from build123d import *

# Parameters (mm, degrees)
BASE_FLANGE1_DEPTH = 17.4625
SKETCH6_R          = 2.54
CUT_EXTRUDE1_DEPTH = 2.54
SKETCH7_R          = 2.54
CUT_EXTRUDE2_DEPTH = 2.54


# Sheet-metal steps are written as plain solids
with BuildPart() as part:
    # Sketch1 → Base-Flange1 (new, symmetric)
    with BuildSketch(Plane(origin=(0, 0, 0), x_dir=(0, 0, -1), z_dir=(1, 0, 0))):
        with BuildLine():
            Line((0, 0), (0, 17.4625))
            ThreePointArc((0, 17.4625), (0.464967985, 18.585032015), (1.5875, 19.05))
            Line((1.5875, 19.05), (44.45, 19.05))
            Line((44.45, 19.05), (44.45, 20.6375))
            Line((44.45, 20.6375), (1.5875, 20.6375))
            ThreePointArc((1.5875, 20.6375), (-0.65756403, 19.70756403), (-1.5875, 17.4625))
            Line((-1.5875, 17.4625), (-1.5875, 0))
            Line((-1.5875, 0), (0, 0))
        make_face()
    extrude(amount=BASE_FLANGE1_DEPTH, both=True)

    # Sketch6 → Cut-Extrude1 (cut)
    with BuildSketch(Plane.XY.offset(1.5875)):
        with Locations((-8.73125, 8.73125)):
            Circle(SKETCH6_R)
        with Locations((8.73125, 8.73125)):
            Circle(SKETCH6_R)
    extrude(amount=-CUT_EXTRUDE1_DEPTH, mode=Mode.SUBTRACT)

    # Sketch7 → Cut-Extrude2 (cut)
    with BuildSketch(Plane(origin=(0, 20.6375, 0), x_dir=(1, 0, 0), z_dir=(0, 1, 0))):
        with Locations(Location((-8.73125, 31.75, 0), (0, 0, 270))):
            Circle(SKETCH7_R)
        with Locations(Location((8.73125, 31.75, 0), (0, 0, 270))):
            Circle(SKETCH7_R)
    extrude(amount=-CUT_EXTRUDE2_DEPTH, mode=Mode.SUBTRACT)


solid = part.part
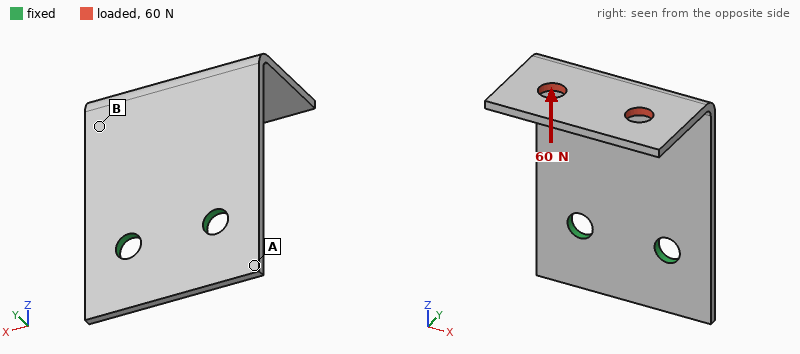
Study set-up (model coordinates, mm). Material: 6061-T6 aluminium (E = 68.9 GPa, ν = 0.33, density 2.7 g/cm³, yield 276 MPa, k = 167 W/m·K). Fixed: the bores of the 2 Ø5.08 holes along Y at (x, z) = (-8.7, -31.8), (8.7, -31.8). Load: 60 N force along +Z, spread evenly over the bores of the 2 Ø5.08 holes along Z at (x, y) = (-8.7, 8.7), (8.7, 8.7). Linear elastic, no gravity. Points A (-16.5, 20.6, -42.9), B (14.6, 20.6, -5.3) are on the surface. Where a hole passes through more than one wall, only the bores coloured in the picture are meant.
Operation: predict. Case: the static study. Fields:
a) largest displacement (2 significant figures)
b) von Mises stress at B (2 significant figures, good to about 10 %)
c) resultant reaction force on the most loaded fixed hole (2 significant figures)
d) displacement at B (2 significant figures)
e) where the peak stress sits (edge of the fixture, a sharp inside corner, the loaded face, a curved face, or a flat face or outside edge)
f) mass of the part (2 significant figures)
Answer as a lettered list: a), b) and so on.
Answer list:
a) 0.67 mm
b) 43 MPa
c) 30 N
d) 0.24 mm
e) a flat face or outside edge
f) 9.2 g
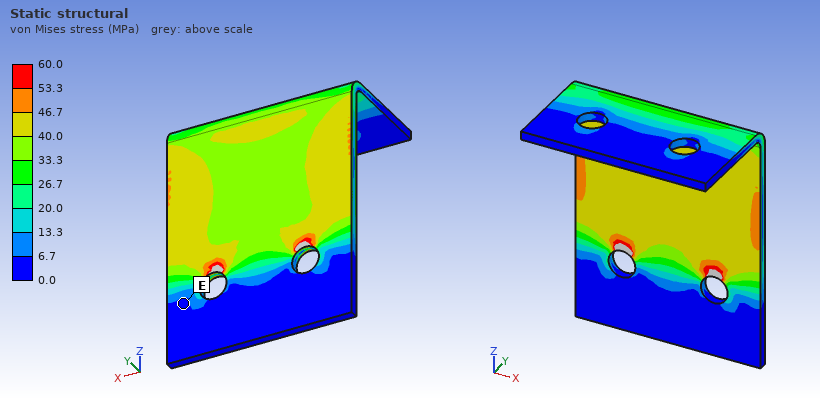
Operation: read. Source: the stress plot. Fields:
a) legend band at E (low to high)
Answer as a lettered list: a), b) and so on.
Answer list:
a) 0.0 to 6.7 MPa
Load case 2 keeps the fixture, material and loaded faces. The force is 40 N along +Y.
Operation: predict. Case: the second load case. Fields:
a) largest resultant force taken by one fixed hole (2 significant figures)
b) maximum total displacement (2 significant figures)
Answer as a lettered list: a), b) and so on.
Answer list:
a) 20 N
b) 0.66 mm
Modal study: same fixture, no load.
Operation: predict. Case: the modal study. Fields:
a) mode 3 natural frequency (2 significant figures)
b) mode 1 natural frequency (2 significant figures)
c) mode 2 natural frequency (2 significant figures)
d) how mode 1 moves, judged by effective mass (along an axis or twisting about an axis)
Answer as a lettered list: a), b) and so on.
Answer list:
a) 2300 Hz
b) 680 Hz
c) 1400 Hz
d) along Y
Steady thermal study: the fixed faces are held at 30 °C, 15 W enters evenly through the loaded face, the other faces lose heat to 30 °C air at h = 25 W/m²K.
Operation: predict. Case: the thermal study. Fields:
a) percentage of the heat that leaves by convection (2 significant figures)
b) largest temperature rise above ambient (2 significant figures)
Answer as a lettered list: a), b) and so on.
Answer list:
a) 21 %
b) 63 K
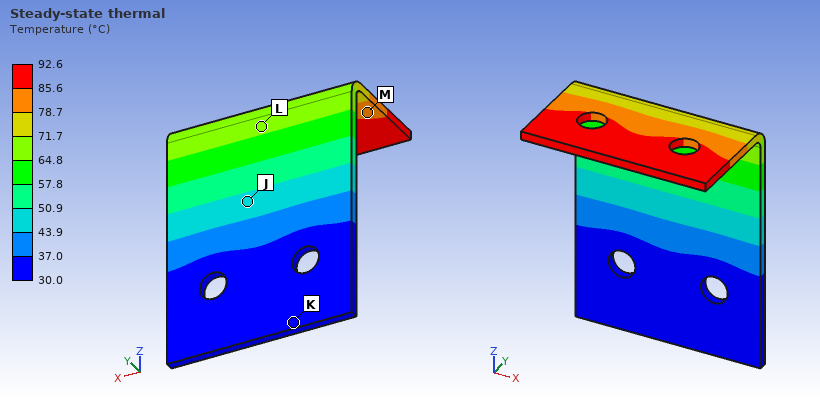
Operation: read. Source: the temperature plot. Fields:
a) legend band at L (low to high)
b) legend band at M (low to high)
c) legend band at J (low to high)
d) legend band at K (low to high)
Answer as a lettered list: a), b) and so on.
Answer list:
a) 64.8 to 71.7 °C
b) 78.7 to 85.6 °C
c) 43.9 to 50.9 °C
d) 30.0 to 37.0 °C
